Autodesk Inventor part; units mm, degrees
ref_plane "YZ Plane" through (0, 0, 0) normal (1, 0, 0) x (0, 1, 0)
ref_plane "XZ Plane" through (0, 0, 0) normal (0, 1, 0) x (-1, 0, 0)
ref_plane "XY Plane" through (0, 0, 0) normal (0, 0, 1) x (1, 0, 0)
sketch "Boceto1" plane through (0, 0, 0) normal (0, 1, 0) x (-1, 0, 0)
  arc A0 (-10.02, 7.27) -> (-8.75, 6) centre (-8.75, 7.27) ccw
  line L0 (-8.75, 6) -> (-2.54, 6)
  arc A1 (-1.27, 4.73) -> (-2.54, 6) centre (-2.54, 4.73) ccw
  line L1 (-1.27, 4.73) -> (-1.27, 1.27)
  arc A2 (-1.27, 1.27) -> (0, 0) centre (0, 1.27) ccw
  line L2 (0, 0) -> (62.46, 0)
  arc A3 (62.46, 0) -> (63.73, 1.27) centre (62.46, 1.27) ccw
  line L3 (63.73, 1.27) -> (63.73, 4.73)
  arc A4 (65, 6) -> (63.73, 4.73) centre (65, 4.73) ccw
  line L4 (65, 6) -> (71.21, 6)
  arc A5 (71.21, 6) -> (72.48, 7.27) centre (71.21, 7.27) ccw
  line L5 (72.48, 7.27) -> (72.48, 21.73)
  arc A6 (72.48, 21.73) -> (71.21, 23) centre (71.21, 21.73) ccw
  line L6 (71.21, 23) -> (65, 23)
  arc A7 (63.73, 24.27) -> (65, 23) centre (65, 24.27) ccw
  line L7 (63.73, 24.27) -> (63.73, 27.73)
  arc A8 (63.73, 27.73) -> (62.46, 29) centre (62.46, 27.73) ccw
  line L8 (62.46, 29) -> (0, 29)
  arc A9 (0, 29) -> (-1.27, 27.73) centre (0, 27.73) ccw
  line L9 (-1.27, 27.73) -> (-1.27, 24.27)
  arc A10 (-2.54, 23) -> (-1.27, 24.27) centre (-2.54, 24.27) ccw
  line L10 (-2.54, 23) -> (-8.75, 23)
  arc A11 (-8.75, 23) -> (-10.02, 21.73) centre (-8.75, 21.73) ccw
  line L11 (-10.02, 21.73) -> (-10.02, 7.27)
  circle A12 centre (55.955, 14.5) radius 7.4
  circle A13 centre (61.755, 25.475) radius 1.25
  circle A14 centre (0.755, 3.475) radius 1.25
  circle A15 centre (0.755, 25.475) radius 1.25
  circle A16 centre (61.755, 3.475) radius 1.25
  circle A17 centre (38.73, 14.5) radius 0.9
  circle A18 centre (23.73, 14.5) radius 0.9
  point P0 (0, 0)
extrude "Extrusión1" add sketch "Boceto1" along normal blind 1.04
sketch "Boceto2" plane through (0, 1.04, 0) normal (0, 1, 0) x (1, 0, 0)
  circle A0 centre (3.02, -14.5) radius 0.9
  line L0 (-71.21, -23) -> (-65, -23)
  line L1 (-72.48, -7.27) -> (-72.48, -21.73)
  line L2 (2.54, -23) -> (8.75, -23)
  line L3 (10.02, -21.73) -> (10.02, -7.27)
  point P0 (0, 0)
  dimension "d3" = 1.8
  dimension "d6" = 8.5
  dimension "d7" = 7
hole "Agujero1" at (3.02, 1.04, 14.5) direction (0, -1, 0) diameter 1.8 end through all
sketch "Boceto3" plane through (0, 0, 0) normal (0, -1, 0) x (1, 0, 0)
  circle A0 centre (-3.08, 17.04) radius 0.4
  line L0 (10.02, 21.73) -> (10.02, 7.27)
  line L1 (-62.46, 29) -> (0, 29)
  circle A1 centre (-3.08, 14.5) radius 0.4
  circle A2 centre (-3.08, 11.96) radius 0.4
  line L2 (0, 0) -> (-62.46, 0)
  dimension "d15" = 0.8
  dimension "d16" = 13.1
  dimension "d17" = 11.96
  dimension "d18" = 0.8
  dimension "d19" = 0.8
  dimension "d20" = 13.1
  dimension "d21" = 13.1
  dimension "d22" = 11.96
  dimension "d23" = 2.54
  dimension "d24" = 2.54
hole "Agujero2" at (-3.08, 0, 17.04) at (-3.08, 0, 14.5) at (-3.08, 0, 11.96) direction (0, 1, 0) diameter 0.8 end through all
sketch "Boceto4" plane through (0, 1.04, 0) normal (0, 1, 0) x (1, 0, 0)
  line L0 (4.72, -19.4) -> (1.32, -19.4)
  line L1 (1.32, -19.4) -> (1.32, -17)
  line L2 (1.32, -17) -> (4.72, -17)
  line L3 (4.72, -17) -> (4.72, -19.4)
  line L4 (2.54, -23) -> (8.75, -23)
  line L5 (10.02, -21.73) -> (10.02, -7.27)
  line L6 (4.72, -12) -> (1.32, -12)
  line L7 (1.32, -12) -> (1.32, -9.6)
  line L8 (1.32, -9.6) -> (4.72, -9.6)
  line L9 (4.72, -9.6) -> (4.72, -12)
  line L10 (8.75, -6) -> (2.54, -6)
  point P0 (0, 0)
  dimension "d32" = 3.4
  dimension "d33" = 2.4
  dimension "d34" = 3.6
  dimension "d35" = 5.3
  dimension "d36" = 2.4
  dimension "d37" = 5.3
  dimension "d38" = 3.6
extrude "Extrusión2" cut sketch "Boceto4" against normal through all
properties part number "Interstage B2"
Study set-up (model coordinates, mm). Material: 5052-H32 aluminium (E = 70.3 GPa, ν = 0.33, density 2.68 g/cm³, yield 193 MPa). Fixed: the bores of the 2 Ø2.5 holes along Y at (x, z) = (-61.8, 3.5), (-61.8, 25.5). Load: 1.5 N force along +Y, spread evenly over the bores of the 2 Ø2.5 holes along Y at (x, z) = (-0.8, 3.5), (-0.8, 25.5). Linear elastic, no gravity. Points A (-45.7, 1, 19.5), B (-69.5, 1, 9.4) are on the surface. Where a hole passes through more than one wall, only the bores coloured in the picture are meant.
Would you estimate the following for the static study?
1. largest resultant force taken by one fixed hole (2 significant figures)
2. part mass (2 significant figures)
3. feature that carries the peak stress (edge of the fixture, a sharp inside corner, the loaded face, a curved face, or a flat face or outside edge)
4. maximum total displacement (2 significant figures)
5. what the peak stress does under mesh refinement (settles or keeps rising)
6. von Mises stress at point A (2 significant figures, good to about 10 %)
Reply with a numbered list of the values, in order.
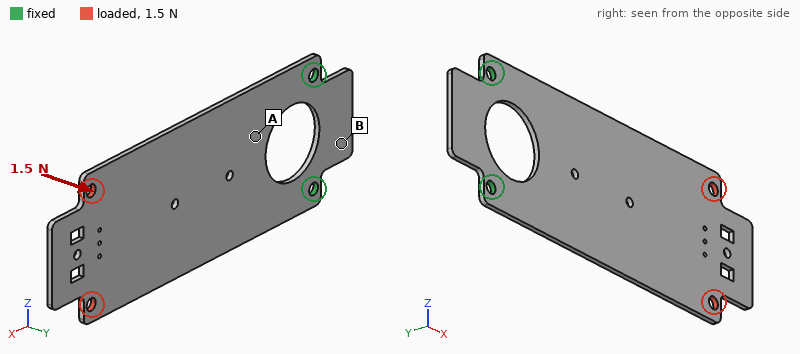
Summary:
1. 0.75 N
2. 5.5 g
3. edge of the fixture
4. 1.0 mm
5. keeps rising
6. 12 MPa
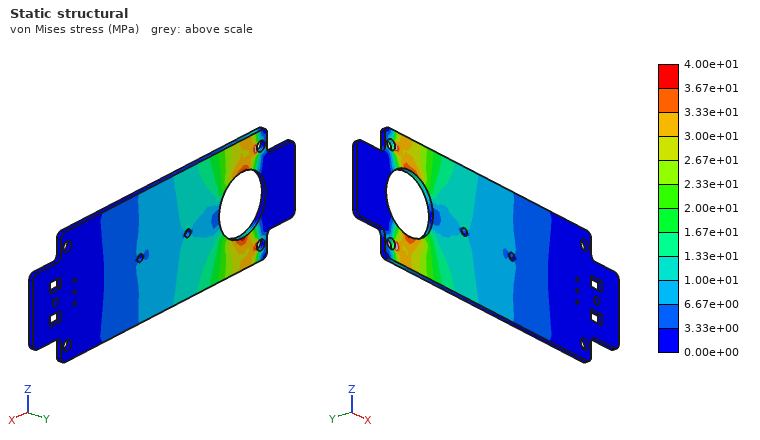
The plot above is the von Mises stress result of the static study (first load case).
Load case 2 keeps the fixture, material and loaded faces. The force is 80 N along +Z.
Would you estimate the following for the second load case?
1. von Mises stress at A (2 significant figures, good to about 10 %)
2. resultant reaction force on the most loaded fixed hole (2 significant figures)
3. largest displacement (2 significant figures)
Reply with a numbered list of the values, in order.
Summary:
1. 12 MPa
2. 210 N
3. 67 µm
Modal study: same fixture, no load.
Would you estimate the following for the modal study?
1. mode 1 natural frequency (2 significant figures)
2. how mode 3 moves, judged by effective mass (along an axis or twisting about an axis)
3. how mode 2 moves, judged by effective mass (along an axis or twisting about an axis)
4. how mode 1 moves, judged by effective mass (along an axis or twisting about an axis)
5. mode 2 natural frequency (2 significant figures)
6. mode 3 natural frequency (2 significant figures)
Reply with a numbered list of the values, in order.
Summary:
1. 160 Hz
2. along Y
3. twisting about X
4. along Y
5. 950 Hz
6. 1100 Hz
